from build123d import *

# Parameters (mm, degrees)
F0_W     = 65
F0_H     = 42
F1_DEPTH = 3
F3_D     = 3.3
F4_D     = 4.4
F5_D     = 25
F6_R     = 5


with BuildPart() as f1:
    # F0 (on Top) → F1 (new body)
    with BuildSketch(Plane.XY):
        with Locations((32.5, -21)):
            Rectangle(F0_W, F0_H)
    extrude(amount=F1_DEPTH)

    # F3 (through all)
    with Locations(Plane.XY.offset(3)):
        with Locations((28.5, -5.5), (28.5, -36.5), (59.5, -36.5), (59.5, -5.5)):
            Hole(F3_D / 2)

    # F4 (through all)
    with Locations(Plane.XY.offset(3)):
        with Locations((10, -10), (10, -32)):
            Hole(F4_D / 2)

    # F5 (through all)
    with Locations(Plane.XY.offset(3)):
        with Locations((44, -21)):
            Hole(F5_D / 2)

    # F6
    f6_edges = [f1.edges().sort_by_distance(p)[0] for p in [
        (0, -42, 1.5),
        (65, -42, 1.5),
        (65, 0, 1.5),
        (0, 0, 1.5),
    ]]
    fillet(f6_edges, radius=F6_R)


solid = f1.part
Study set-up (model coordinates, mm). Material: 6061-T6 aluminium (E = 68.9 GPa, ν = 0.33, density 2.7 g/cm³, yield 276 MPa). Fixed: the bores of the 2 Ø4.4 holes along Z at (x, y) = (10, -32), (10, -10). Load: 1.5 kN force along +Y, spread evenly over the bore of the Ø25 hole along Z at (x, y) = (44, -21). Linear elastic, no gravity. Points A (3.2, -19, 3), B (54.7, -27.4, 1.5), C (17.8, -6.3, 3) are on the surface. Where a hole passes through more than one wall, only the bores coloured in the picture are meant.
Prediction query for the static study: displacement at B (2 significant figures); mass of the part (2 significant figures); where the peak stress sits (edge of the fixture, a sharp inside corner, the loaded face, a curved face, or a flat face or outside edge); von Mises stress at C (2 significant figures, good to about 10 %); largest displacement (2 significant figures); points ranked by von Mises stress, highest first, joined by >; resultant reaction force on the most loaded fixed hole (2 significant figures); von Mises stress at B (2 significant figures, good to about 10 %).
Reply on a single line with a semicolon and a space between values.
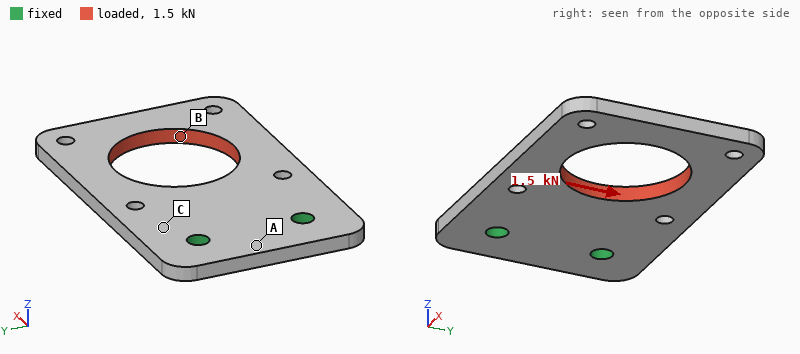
0.10 mm; 17 g; edge of the fixture; 32 MPa; 0.12 mm; B > C > A; 2.2 kN; 56 MPa
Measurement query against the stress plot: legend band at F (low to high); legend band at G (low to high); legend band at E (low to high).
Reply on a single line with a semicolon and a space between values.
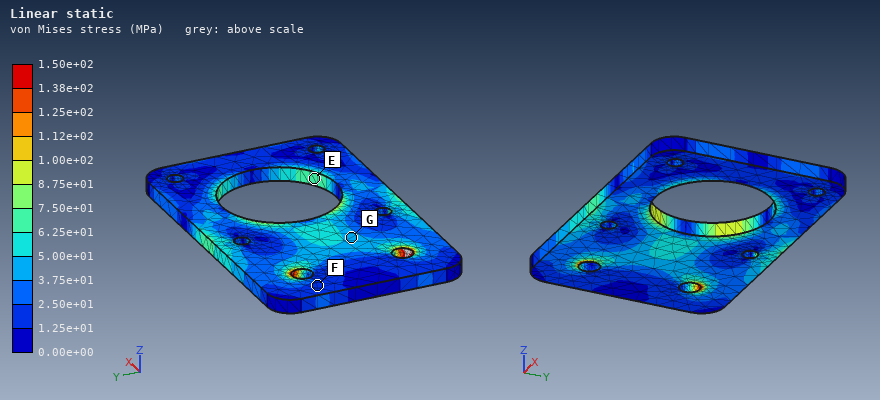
1.25e+01 to 2.50e+01 MPa; 3.75e+01 to 5.00e+01 MPa; 6.25e+01 to 7.50e+01 MPa
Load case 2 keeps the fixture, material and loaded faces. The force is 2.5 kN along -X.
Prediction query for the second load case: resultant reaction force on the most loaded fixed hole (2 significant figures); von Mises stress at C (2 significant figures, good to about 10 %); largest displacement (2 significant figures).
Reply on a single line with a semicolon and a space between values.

1.3 kN; 27 MPa; 35 µm
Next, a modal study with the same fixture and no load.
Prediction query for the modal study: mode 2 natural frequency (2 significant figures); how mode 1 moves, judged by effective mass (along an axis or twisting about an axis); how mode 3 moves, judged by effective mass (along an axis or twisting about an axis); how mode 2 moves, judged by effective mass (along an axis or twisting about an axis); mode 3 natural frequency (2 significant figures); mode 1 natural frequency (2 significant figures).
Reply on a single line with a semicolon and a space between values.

2200 Hz; along Z; along Z; twisting about X; 4700 Hz; 870 Hz
